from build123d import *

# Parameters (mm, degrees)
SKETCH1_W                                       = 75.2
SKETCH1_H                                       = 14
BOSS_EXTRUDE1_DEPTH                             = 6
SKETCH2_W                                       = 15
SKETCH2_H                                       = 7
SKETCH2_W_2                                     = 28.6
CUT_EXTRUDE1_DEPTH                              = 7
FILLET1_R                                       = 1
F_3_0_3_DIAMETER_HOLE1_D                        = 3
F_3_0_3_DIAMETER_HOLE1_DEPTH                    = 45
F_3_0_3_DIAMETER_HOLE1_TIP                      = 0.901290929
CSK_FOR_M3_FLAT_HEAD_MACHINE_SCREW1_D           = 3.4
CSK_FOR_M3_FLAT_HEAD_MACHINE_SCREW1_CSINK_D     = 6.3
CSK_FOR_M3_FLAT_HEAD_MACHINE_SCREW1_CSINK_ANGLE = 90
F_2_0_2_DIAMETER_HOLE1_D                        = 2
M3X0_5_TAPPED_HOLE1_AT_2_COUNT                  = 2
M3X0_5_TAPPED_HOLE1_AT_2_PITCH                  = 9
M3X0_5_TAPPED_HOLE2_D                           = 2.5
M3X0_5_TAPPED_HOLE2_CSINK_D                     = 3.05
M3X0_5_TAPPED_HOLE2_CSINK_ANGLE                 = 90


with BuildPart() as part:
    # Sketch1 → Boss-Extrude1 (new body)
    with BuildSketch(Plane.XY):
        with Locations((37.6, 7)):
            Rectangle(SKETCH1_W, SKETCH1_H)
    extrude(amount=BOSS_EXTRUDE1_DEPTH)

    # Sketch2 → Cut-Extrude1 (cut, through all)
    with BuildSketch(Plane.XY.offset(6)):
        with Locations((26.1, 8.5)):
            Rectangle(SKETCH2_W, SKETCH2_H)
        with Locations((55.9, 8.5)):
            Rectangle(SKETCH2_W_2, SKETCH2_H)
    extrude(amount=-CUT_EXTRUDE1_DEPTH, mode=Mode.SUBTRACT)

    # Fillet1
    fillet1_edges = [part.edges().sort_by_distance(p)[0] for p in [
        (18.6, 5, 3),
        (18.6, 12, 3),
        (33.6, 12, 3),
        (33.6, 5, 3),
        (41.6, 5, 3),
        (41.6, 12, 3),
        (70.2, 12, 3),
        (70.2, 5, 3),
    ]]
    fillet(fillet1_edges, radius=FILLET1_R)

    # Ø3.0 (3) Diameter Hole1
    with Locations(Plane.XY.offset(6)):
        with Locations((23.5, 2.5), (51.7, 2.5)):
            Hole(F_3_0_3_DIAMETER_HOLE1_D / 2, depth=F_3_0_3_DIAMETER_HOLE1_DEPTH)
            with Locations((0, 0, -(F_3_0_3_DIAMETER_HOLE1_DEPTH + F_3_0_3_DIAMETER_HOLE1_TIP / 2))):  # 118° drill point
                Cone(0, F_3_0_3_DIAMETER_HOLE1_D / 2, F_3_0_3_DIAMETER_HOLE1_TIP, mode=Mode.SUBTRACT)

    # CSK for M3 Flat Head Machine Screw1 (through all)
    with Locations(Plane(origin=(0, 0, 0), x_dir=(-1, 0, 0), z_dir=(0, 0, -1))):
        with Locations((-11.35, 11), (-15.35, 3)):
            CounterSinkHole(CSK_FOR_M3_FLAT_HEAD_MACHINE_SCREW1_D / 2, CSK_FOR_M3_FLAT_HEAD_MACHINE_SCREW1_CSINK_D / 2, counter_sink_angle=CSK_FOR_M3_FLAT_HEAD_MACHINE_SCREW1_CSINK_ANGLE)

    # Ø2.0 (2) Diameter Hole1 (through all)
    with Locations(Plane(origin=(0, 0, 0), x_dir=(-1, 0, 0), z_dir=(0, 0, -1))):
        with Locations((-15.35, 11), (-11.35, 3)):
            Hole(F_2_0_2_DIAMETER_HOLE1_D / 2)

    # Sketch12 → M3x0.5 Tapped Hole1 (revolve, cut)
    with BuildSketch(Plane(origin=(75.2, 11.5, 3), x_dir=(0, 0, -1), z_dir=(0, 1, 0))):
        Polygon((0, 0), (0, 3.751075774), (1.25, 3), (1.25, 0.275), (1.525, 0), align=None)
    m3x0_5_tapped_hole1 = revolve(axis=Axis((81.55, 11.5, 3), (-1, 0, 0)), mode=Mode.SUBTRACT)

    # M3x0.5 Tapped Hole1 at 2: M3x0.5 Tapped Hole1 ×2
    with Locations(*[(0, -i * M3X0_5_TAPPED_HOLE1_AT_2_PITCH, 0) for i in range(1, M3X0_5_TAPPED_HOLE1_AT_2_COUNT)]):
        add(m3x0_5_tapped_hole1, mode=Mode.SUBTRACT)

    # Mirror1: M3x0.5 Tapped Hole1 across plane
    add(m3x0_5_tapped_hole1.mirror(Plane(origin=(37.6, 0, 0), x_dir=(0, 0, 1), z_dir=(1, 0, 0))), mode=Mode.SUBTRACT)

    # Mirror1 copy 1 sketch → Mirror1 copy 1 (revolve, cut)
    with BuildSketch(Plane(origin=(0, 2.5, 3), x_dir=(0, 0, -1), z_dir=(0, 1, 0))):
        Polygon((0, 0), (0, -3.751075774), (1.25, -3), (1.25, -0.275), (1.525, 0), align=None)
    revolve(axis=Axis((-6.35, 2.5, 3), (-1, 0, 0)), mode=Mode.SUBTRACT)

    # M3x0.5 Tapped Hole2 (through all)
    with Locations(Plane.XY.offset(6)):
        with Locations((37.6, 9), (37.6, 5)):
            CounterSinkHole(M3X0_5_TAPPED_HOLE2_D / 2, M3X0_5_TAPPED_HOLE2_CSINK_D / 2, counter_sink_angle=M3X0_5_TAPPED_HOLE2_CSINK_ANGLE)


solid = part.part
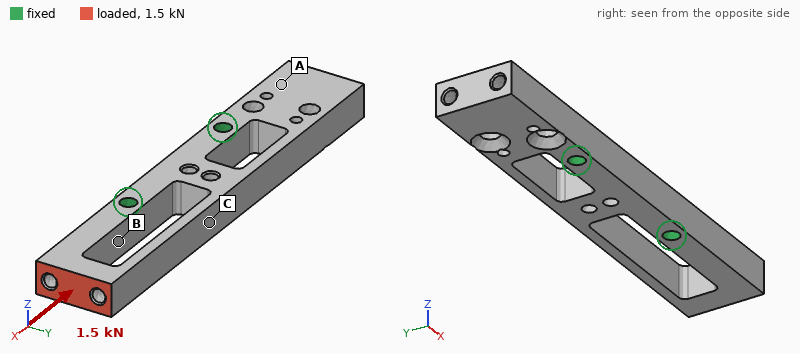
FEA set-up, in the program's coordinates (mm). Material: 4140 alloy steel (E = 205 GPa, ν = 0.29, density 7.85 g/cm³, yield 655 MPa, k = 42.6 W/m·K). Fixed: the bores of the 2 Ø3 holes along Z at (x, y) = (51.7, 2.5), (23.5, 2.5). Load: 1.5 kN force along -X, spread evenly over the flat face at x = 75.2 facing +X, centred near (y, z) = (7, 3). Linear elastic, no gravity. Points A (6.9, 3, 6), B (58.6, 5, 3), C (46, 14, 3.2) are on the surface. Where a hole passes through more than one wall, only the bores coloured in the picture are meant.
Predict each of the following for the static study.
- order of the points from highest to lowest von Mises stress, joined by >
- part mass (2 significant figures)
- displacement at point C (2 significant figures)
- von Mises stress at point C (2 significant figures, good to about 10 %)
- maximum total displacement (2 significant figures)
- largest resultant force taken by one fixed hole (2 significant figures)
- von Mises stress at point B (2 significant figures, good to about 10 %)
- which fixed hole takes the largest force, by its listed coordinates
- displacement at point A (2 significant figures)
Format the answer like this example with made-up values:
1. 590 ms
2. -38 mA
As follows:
1. B > C > A
2. 32 g
3. 11 µm
4. 34 MPa
5. 23 µm
6. 1.2 kN
7. 69 MPa
8. (51.7, 2.5)
9. 7.2 µm
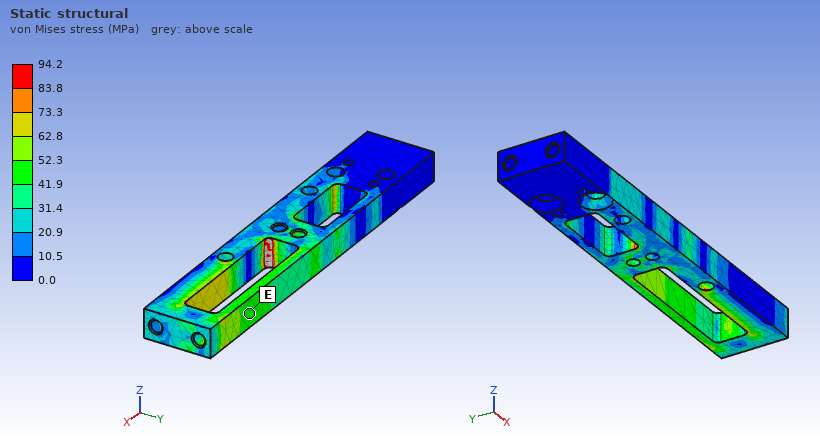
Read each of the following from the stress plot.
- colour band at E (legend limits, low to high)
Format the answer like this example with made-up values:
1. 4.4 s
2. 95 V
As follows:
1. 41.9 to 52.3 MPa
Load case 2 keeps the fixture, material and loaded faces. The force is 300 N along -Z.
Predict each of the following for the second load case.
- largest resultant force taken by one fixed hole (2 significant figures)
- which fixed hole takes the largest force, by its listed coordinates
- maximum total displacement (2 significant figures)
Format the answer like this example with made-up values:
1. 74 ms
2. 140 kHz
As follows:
1. 340 N
2. (51.7, 2.5)
3. 82 µm
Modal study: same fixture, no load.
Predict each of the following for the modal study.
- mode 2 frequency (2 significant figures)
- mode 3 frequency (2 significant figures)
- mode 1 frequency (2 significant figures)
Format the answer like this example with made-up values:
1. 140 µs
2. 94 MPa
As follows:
1. 5600 Hz
2. 6600 Hz
3. 5500 Hz
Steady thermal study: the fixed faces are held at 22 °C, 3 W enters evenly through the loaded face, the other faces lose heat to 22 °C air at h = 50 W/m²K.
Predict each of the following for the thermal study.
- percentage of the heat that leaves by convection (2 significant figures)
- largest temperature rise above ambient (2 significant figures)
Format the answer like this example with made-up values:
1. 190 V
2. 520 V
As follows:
1. 35 %
2. 32 K
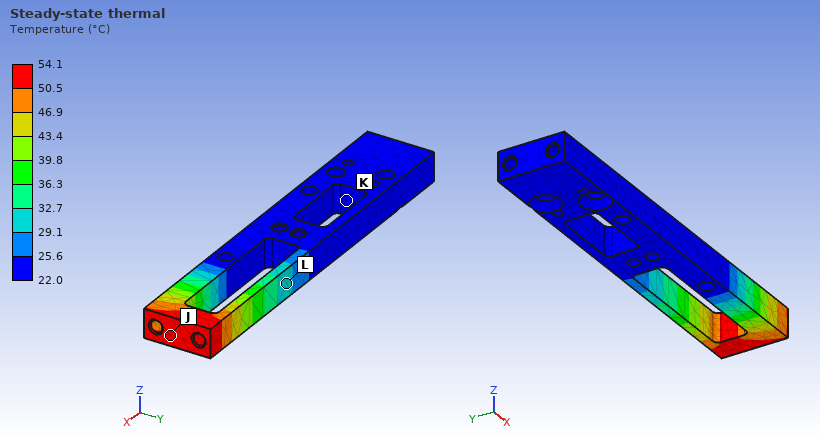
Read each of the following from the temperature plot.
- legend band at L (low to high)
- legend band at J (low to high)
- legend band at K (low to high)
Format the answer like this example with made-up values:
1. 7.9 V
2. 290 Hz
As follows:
1. 29.1 to 32.7 °C
2. 50.5 to 54.1 °C
3. 22.0 to 25.6 °C
